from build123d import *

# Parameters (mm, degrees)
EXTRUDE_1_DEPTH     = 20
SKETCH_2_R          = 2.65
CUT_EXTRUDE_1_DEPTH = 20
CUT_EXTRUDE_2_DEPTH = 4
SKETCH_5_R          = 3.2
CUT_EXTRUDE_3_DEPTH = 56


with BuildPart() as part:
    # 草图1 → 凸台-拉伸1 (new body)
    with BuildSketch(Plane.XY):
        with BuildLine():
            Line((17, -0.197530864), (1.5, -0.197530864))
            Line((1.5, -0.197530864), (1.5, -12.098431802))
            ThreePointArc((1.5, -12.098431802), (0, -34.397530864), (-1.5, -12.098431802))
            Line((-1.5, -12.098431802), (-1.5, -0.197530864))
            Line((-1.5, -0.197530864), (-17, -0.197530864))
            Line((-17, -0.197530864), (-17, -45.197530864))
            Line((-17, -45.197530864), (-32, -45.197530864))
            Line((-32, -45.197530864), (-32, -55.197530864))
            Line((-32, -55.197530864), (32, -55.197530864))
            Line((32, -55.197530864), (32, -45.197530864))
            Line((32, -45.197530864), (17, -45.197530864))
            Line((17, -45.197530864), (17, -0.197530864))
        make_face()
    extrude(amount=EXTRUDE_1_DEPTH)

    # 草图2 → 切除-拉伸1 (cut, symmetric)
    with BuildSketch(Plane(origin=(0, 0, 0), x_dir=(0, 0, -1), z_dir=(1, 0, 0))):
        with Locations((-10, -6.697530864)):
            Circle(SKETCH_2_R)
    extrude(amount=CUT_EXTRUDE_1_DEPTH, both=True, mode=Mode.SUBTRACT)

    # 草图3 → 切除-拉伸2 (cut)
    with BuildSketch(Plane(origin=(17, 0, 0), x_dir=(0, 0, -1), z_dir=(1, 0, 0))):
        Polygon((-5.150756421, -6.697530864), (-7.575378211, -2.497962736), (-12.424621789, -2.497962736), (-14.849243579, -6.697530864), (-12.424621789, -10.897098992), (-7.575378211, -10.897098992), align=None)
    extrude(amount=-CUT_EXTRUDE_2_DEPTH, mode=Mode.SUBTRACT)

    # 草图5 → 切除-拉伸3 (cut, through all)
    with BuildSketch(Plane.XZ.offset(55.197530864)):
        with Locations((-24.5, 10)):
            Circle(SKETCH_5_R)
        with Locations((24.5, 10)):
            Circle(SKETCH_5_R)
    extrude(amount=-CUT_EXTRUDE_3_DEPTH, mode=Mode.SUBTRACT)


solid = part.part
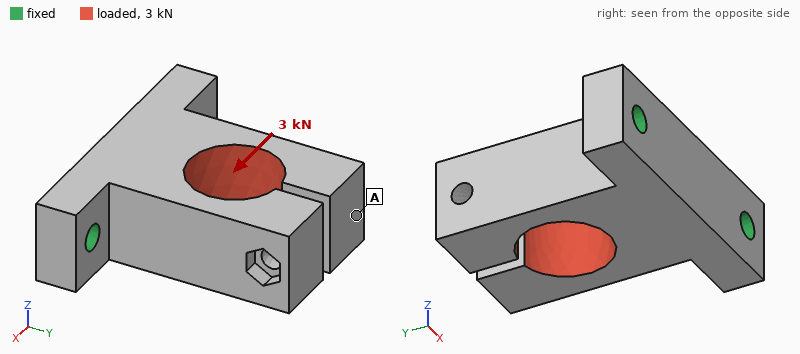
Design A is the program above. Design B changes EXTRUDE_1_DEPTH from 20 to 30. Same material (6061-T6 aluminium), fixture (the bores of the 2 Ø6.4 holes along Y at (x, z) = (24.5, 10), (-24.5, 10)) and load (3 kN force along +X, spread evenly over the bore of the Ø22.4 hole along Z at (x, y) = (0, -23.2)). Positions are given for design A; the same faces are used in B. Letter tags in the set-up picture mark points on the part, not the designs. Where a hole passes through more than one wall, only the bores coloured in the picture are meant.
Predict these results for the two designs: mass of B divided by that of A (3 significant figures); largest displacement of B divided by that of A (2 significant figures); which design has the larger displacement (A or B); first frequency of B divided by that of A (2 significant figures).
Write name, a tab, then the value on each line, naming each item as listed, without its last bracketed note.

mass of B divided by that of A	1.52
largest displacement of B divided by that of A	0.68
which design has the larger displacement	A
first frequency of B divided by that of A	0.97
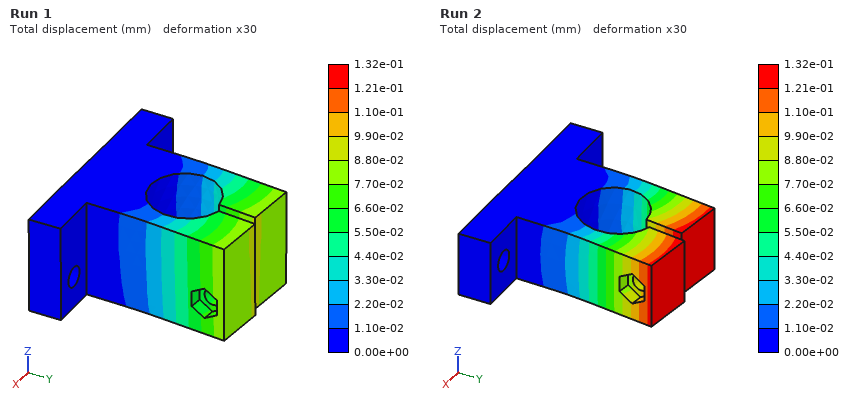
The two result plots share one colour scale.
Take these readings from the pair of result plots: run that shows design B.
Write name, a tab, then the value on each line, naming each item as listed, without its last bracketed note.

run that shows design B	Run 1
